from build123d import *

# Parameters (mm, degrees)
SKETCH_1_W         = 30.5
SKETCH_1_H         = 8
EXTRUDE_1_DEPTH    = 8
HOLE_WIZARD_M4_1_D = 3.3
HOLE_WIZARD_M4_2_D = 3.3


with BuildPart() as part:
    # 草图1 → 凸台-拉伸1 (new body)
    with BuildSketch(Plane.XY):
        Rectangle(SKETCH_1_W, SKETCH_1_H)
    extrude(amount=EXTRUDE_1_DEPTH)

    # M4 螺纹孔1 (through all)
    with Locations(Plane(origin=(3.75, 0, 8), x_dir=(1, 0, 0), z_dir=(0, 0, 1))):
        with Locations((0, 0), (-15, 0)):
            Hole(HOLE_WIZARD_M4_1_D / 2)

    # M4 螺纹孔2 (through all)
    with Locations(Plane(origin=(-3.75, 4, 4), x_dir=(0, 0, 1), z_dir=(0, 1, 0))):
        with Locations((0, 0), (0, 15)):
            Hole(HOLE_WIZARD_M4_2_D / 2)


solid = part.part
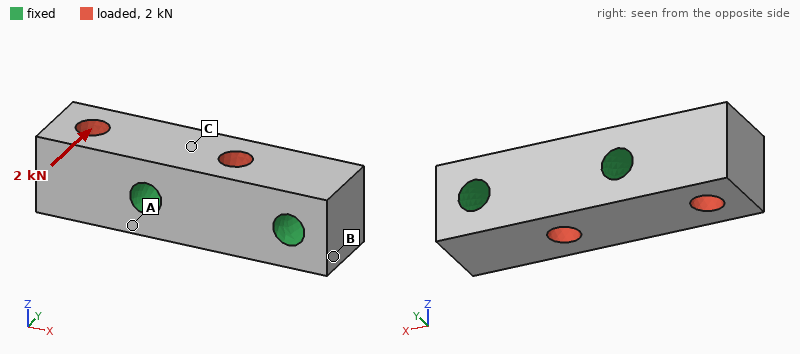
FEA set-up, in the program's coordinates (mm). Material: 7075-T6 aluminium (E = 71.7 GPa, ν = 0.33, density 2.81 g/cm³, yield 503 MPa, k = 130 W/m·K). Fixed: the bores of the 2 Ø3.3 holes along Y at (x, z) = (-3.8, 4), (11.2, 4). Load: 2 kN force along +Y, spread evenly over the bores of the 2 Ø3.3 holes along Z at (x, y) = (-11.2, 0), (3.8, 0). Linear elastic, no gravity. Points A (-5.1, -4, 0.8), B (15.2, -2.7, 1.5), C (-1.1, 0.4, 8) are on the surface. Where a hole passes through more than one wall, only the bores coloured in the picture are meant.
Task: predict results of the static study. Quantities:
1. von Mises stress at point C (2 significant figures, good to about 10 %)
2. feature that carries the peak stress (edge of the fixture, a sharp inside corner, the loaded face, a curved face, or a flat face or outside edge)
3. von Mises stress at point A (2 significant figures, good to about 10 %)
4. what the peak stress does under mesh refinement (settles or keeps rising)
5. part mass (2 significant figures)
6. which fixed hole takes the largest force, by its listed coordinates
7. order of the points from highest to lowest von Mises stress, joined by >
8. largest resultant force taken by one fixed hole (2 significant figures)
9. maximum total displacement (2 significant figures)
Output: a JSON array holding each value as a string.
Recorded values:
["19 MPa", "edge of the fixture", "47 MPa", "keeps rising", "4.7 g", "(-3.8, 4)", "A > C > B", "1.5 kN", "16 µm"]
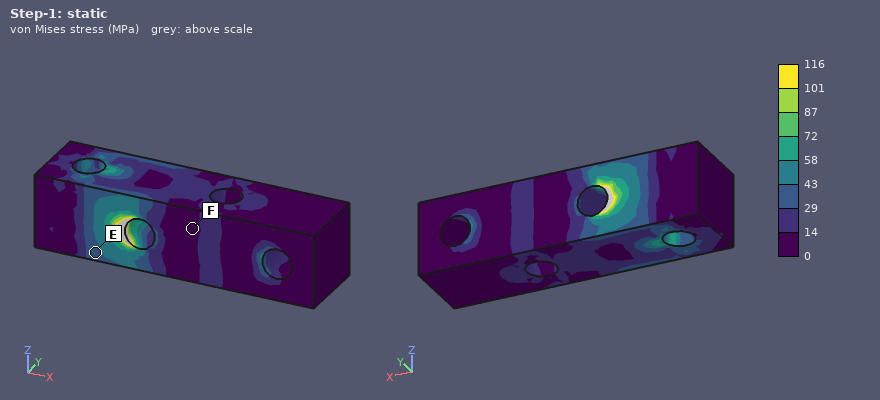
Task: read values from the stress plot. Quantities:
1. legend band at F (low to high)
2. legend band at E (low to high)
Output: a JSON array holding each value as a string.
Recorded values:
["0 to 14 MPa", "29 to 43 MPa"]
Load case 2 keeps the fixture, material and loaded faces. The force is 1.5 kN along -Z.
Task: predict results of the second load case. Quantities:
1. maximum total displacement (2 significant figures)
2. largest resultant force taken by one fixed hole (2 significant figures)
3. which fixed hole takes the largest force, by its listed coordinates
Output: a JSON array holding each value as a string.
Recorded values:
["15 µm", "1.2 kN", "(-3.8, 4)"]
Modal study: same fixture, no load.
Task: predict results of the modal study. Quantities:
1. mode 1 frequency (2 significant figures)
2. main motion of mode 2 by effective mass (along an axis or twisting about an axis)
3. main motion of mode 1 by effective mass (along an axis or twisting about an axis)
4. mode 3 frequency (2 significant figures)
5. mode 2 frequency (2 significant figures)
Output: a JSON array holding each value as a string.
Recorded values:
["35 kHz", "along Y", "along Z", "63 kHz", "40 kHz"]
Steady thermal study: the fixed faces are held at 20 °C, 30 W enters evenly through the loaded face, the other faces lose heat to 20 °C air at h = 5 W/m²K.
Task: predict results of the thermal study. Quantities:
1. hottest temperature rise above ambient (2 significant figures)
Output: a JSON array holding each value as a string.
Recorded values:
["16 K"]
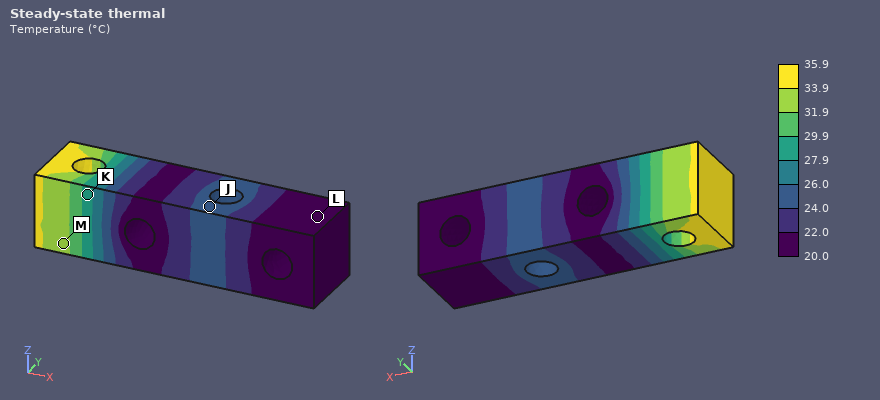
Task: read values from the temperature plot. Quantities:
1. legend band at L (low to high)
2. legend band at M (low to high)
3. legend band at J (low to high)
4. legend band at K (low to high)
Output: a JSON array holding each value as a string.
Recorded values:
["20.0 to 22.0 °C", "31.9 to 33.9 °C", "24.0 to 26.0 °C", "27.9 to 29.9 °C"]
